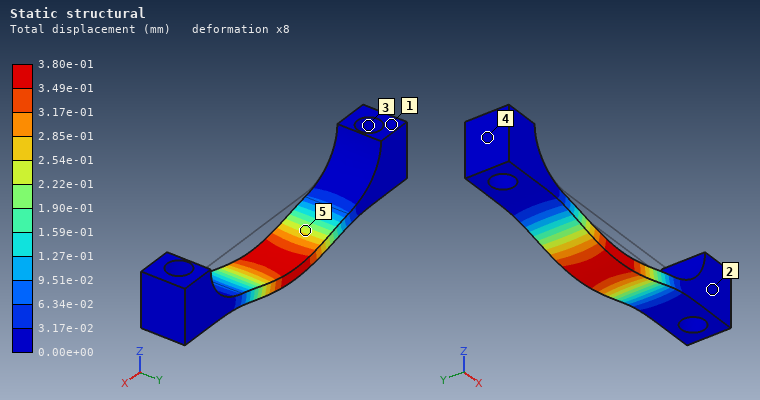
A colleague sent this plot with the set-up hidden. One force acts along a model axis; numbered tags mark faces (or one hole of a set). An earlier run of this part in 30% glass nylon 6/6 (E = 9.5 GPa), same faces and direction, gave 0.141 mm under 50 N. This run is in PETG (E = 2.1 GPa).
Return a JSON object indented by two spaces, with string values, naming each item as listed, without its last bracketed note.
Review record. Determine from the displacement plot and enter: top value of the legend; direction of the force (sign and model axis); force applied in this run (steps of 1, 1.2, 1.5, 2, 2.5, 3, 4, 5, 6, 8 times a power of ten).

{
  "top value of the legend": "3.80e-01 mm",
  "direction of the force": "-Z",
  "force applied in this run": "30 N"
}
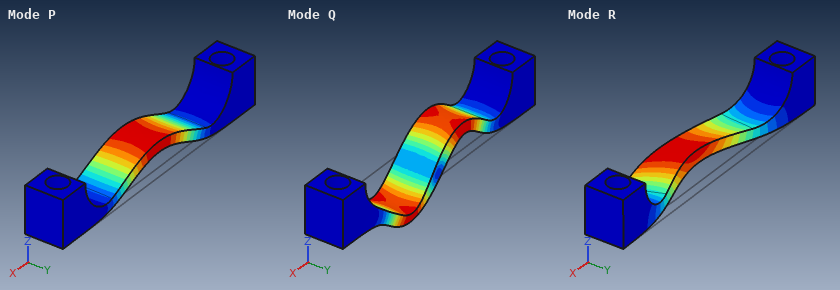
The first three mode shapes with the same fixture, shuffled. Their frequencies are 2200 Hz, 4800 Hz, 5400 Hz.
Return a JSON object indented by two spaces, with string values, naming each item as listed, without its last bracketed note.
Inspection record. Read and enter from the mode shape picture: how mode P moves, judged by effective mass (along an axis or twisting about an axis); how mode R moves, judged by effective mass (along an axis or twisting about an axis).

{
  "how mode P moves, judged by effective mass": "along Z",
  "how mode R moves, judged by effective mass": "along Y"
}
